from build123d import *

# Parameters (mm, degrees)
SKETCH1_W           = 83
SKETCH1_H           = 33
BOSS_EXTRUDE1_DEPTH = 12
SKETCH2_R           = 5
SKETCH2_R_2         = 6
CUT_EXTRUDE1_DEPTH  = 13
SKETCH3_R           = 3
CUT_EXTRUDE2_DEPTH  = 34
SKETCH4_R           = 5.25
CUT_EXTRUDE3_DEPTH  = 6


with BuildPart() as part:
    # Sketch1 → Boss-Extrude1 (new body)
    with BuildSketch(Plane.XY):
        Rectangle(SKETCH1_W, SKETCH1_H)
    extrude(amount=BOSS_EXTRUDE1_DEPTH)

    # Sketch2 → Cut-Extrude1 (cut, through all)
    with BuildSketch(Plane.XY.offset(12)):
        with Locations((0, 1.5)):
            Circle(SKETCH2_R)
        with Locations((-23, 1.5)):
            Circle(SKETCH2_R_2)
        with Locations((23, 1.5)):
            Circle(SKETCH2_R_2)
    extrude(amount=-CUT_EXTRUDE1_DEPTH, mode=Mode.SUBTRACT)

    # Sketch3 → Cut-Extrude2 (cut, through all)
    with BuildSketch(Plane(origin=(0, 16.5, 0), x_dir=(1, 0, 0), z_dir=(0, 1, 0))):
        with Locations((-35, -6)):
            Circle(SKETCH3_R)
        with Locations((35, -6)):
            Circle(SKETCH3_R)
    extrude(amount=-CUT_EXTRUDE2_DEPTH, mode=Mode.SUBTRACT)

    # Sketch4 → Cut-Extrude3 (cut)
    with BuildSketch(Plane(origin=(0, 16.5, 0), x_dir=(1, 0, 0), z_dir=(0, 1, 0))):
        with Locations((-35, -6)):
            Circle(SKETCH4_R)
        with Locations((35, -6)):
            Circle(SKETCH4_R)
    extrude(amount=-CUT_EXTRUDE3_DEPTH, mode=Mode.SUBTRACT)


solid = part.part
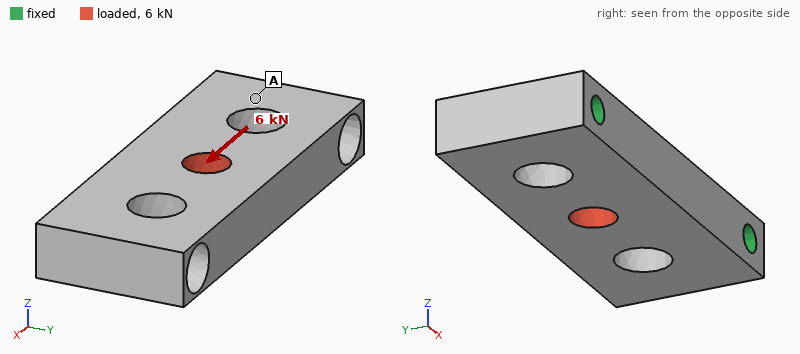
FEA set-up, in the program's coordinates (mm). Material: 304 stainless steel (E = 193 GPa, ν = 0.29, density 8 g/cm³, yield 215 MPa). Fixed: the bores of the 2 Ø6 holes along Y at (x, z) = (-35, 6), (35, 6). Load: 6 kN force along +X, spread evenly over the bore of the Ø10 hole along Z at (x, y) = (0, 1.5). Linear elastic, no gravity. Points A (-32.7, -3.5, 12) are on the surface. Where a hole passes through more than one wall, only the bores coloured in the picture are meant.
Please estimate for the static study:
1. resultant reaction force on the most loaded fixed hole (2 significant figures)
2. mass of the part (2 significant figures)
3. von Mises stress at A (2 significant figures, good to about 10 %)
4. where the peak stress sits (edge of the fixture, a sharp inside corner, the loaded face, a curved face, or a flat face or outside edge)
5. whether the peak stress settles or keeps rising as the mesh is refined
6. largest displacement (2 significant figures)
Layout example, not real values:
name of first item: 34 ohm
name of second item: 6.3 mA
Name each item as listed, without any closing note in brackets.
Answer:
resultant reaction force on the most loaded fixed hole: 3.0 kN
mass of the part: 210 g
von Mises stress at A: 4.1 MPa
where the peak stress sits: edge of the fixture
whether the peak stress settles or keeps rising as the mesh is refined: keeps rising
largest displacement: 2.6 µm
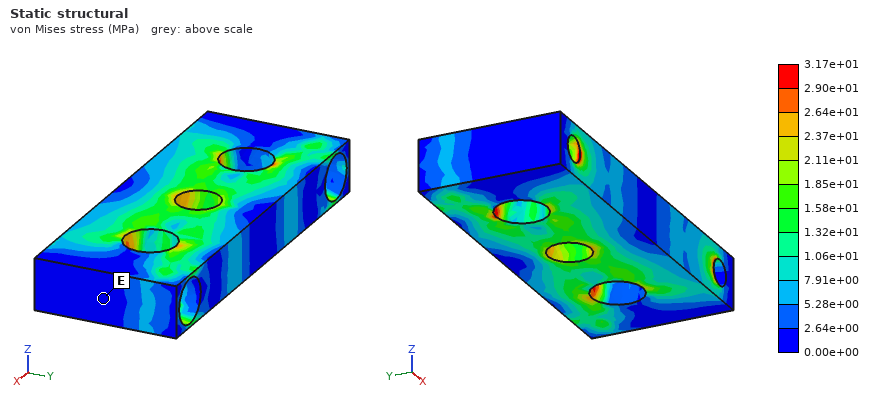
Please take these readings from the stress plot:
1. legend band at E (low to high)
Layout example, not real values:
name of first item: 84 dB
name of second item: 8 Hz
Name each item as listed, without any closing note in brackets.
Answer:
legend band at E: 0.00e+00 to 2.64e+00 MPa
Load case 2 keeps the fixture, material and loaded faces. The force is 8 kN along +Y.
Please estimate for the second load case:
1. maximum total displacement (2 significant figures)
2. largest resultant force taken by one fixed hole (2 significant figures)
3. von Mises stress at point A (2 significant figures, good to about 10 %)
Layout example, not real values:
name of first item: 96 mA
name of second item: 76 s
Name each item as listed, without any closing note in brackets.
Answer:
maximum total displacement: 12 µm
largest resultant force taken by one fixed hole: 4.2 kN
von Mises stress at point A: 20 MPa
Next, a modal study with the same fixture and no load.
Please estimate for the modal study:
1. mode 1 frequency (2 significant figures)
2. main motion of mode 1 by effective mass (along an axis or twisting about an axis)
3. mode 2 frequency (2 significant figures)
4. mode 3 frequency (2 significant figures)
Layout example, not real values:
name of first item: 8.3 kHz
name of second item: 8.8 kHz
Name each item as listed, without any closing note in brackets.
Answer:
mode 1 frequency: 9300 Hz
main motion of mode 1 by effective mass: along Z
mode 2 frequency: 13 kHz
mode 3 frequency: 14 kHz
